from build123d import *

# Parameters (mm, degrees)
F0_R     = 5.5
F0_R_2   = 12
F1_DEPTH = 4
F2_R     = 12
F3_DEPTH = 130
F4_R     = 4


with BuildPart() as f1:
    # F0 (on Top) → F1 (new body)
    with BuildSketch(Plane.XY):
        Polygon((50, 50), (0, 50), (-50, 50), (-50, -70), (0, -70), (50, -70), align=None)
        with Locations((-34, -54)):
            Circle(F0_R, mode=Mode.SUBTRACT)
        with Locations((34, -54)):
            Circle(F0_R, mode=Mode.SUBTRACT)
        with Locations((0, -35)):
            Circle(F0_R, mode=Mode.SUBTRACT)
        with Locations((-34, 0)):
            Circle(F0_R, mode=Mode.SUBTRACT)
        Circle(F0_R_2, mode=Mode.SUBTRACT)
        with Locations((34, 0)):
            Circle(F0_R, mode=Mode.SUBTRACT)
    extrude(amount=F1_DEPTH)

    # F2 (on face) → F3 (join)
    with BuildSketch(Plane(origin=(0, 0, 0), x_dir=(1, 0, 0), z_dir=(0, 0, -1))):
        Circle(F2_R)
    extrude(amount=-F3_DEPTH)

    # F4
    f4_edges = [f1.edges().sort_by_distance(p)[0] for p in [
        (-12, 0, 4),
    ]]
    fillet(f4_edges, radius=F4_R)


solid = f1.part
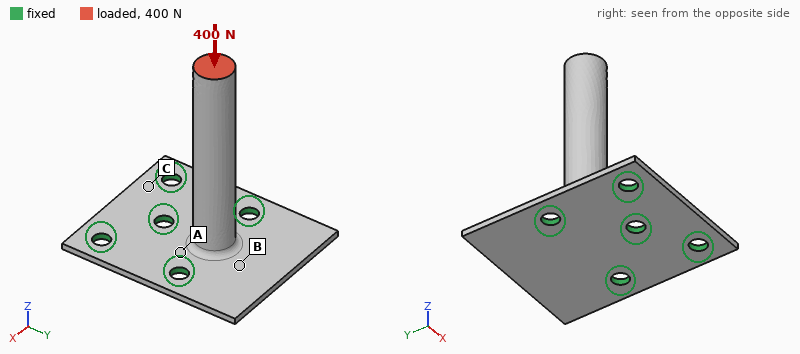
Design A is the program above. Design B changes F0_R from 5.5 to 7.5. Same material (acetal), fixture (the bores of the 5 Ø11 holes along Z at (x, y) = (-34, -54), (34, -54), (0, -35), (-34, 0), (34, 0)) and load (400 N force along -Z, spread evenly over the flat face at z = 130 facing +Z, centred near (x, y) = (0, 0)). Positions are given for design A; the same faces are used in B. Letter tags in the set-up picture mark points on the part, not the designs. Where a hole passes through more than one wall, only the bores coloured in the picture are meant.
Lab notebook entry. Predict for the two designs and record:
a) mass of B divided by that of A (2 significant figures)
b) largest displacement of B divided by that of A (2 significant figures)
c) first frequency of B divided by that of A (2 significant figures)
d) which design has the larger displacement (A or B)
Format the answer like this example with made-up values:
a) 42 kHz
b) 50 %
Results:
a) 0.98
b) 0.76
c) 1.1
d) A
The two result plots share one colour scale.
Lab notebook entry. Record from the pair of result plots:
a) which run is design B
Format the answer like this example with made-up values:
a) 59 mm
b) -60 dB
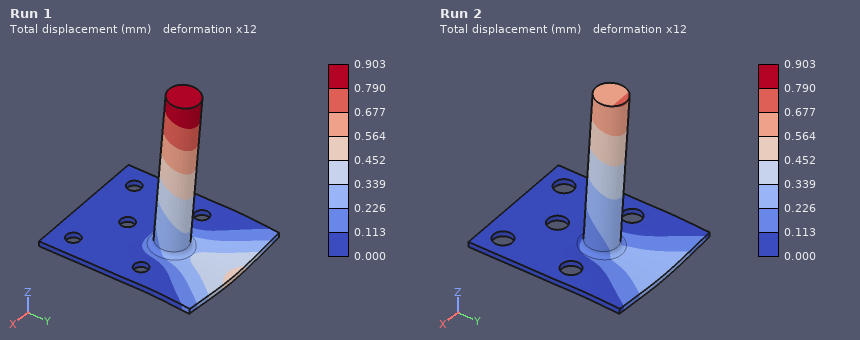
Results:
a) Run 2
